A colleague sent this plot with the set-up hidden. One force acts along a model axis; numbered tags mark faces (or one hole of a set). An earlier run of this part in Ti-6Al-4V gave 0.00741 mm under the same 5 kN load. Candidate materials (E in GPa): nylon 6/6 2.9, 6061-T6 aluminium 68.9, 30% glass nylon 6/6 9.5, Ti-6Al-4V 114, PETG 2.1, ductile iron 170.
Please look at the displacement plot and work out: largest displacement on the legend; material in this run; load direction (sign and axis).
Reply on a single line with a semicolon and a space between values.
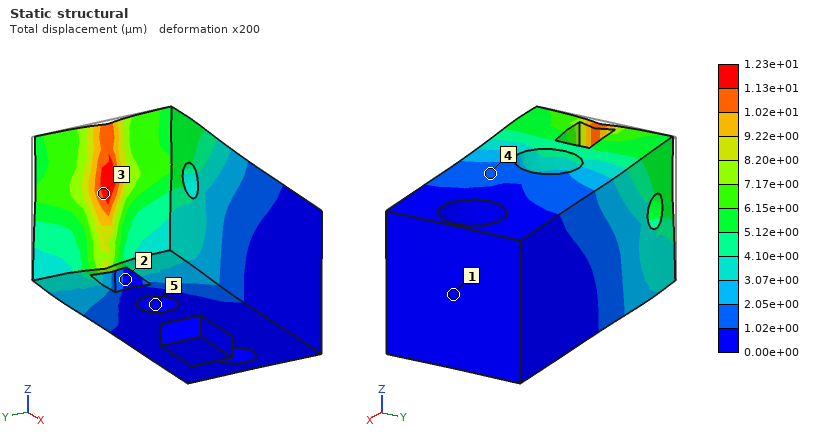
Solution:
1.23e+01 µm; 6061-T6 aluminium; +X
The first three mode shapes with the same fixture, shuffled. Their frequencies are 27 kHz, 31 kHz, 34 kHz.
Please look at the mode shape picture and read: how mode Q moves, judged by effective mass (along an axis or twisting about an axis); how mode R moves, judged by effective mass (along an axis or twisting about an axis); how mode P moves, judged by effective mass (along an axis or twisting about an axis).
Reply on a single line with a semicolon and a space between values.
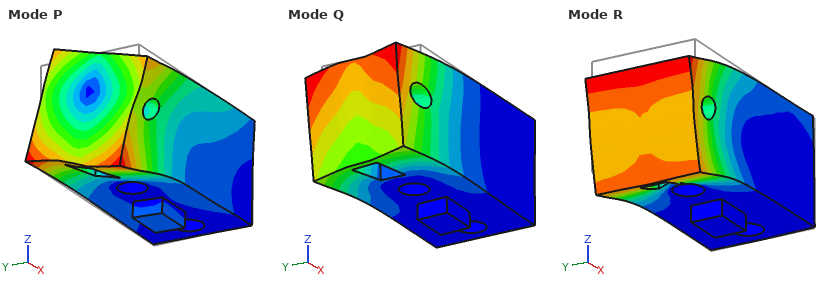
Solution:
along Y; along Z; twisting about X
